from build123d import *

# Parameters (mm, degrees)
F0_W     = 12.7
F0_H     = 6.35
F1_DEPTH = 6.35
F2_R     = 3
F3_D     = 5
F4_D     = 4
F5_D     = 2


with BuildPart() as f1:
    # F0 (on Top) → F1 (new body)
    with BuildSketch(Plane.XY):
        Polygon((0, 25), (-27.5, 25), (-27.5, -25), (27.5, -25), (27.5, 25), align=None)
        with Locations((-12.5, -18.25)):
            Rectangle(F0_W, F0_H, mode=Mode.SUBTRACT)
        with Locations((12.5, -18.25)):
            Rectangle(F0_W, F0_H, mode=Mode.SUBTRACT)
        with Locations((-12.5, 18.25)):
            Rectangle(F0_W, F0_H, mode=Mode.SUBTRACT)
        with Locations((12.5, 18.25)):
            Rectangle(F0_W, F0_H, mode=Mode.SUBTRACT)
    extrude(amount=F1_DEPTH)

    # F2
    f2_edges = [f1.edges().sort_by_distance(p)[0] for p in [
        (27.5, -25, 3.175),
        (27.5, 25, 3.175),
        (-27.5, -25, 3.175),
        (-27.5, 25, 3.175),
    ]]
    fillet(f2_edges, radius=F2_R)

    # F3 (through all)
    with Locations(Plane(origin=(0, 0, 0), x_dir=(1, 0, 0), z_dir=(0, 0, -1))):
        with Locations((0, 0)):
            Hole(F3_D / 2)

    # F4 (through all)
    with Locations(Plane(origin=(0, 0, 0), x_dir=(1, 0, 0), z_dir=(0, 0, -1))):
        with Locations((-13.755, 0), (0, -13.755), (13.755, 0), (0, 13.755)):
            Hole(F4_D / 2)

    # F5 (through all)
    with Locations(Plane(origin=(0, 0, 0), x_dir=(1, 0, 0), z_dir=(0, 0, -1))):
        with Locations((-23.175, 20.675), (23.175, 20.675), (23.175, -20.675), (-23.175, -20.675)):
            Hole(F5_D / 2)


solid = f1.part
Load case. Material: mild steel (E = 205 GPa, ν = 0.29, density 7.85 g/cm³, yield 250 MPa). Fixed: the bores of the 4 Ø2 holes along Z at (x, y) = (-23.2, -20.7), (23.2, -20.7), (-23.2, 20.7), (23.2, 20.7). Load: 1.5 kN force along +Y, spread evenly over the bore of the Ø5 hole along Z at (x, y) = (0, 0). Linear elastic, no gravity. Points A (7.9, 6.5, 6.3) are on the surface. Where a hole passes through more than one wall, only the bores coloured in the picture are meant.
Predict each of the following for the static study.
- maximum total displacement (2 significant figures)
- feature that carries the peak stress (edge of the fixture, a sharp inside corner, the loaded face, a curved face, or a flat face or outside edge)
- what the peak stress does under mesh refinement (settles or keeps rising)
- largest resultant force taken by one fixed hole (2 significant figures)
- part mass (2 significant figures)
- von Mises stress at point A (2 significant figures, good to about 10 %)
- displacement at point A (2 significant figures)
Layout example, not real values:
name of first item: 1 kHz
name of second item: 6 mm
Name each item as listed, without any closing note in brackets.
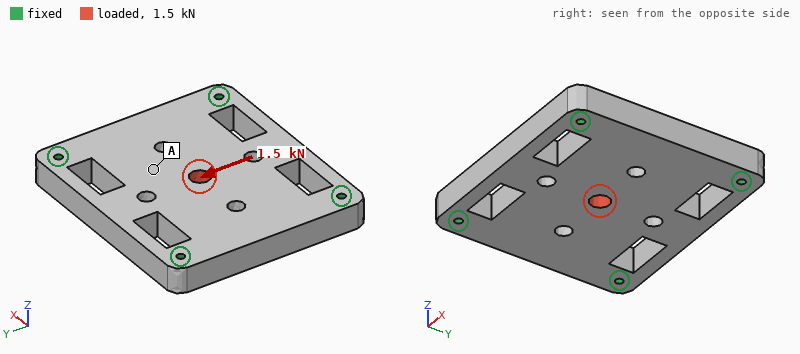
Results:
maximum total displacement: 2.1 µm
feature that carries the peak stress: edge of the fixture
what the peak stress does under mesh refinement: keeps rising
largest resultant force taken by one fixed hole: 420 N
part mass: 120 g
von Mises stress at point A: 7.3 MPa
displacement at point A: 1.4 µm
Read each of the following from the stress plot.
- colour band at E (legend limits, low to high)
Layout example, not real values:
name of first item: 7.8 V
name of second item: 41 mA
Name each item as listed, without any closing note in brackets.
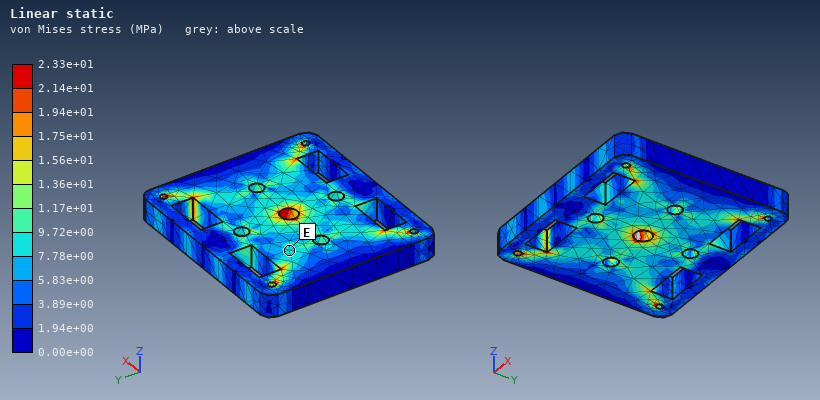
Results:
colour band at E: 7.78e+00 to 9.72e+00 MPa
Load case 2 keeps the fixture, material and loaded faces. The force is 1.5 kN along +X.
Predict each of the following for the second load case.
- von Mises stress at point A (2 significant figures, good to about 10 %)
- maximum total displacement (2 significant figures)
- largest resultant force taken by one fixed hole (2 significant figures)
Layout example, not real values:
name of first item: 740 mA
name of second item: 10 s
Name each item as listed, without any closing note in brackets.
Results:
von Mises stress at point A: 7.6 MPa
maximum total displacement: 1.9 µm
largest resultant force taken by one fixed hole: 400 N
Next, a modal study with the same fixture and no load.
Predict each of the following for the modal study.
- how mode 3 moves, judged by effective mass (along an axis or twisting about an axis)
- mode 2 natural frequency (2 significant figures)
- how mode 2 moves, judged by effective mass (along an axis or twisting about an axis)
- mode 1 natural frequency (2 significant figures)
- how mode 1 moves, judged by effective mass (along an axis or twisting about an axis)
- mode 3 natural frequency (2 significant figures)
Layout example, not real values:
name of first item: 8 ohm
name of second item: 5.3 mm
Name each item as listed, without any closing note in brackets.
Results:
how mode 3 moves, judged by effective mass: twisting about Y
mode 2 natural frequency: 13 kHz
how mode 2 moves, judged by effective mass: twisting about X
mode 1 natural frequency: 8400 Hz
how mode 1 moves, judged by effective mass: along Z
mode 3 natural frequency: 16 kHz
